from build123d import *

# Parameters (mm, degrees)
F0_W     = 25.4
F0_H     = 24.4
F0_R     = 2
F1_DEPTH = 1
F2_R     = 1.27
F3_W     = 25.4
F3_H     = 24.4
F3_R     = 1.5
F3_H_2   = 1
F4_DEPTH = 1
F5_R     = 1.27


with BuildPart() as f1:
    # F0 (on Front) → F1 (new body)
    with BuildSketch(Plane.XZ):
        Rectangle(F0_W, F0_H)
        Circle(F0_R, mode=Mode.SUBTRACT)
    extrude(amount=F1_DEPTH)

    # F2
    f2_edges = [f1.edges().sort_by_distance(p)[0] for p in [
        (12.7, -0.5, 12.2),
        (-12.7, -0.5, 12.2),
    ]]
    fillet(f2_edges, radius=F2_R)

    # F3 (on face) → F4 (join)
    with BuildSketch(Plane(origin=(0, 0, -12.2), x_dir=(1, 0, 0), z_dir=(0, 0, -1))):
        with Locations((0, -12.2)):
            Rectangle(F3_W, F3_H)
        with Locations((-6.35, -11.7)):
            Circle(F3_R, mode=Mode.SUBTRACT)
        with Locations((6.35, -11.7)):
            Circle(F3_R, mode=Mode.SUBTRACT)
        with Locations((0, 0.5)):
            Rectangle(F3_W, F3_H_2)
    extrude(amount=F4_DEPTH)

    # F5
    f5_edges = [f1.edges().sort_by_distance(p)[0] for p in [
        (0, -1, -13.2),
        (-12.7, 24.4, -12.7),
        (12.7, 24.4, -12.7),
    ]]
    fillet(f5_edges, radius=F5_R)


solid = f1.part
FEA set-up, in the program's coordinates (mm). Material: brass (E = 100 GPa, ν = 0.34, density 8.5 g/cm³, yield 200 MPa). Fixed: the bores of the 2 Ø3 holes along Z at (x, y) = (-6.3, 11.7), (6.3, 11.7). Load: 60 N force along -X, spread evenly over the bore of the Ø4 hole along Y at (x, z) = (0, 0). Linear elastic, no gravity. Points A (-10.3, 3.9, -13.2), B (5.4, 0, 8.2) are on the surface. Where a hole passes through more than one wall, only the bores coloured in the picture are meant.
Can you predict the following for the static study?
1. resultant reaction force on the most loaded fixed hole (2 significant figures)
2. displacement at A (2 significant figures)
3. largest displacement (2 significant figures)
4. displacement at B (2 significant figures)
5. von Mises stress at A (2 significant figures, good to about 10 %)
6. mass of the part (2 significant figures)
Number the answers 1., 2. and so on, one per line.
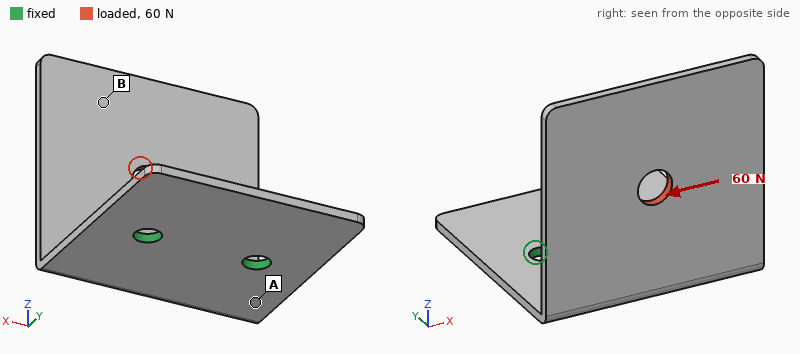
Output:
1. 73 N
2. 0.066 mm
3. 0.32 mm
4. 0.25 mm
5. 57 MPa
6. 10 g
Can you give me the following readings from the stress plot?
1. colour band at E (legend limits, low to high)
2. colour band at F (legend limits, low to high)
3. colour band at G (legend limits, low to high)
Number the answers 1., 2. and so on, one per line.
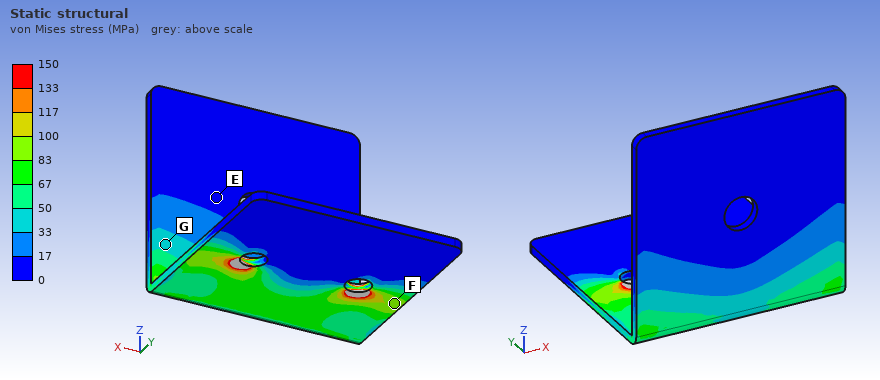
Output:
1. 0 to 17 MPa
2. 83 to 100 MPa
3. 33 to 50 MPa
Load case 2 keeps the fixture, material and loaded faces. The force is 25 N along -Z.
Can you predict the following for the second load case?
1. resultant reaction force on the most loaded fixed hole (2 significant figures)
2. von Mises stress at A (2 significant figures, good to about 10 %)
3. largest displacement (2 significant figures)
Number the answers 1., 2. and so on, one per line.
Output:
1. 13 N
2. 25 MPa
3. 0.19 mm
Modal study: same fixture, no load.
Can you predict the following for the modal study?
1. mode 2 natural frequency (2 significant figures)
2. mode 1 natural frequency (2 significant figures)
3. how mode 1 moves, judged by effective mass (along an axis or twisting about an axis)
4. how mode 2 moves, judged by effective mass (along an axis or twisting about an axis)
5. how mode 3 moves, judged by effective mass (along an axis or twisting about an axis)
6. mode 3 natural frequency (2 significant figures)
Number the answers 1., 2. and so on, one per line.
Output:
1. 1100 Hz
2. 530 Hz
3. along Y
4. along X
5. along Z
6. 1900 Hz
